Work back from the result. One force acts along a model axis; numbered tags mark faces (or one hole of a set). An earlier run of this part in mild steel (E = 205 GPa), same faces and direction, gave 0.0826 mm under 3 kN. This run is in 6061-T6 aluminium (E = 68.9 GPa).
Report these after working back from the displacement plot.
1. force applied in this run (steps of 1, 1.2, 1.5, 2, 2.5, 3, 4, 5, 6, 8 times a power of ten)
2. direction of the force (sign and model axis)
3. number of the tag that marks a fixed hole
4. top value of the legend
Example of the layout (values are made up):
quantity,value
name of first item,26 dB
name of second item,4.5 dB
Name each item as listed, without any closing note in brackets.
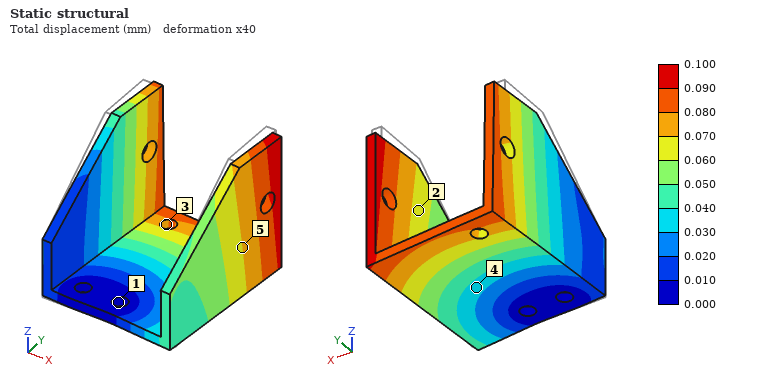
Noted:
quantity,value
force applied in this run,1.2 kN
direction of the force,+X
number of the tag that marks a fixed hole,1
top value of the legend,0.100 mm
